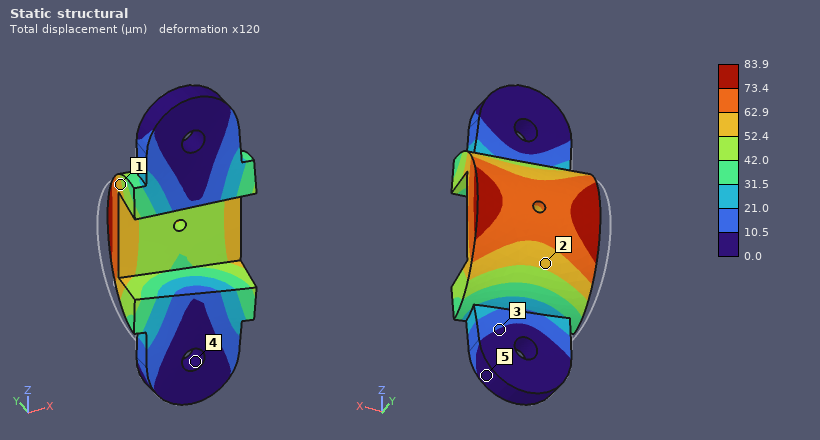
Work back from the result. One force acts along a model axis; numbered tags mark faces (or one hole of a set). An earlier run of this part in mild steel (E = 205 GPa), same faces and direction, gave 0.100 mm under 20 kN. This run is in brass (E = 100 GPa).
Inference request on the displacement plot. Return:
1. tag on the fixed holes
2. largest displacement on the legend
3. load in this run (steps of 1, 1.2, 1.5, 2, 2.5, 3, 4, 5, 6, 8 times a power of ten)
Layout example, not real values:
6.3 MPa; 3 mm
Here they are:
4; 83.9 µm; 8 kN
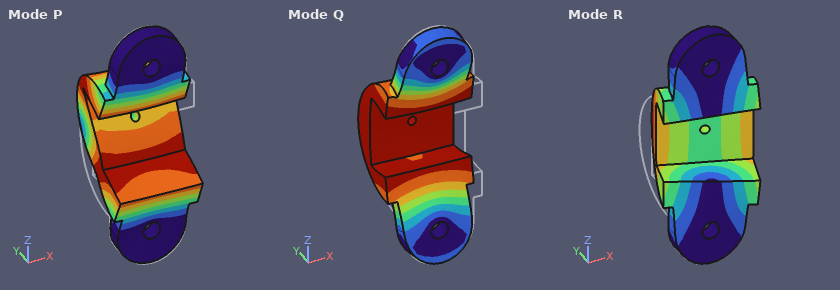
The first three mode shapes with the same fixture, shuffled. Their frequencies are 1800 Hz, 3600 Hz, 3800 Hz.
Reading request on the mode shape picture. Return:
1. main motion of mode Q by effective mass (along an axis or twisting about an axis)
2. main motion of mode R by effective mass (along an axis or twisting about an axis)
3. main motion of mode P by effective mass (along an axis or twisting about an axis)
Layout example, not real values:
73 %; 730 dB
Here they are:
along Y; along X; along Z
